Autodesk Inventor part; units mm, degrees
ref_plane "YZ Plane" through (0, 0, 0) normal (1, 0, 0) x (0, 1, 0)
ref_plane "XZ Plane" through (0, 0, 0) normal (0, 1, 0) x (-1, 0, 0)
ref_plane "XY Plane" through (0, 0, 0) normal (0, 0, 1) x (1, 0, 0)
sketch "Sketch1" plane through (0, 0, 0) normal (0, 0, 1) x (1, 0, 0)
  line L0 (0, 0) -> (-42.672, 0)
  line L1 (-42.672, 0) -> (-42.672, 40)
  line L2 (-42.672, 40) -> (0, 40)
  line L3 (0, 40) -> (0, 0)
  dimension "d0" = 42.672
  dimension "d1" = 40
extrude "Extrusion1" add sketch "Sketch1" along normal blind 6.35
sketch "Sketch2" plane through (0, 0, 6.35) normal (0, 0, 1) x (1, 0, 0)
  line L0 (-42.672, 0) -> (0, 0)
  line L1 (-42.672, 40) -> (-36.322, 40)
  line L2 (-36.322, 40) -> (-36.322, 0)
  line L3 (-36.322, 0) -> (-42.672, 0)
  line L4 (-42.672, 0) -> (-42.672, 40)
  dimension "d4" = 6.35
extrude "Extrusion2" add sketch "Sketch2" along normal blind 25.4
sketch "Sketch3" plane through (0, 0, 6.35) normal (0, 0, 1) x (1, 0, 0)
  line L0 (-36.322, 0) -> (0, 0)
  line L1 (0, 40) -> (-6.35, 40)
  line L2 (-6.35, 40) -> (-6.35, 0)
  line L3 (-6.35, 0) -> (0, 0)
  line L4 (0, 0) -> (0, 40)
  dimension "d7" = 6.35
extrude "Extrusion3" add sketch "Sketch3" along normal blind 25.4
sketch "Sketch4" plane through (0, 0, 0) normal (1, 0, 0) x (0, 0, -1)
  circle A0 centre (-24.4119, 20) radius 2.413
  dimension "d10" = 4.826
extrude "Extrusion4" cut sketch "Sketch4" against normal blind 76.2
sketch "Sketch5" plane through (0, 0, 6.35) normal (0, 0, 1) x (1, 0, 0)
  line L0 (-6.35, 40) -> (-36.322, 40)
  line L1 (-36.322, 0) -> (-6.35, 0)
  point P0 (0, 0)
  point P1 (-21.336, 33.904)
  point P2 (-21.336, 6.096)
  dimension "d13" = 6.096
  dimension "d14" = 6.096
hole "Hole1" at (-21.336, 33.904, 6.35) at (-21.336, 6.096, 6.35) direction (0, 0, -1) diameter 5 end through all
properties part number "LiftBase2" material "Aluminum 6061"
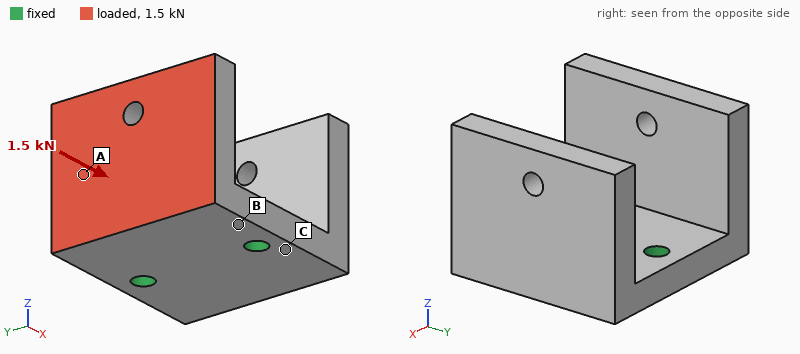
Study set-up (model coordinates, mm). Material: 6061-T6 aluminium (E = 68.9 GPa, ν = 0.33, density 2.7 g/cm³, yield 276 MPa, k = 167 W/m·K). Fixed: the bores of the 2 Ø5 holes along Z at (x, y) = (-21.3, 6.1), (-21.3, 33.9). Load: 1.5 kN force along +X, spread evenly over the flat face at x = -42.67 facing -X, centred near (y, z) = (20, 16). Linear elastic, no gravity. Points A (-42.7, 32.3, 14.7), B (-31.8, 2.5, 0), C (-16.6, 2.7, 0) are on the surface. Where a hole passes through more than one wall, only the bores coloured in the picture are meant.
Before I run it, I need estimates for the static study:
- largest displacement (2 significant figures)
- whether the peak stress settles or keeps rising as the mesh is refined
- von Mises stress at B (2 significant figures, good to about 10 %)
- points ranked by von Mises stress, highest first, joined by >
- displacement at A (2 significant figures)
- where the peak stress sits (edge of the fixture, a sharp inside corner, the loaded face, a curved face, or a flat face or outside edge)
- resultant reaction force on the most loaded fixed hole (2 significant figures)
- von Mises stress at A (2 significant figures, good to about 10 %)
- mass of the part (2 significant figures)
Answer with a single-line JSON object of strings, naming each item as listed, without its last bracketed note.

{"largest displacement": "0.22 mm", "whether the peak stress settles or keeps rising as the mesh is refined": "keeps rising", "von Mises stress at B": "68 MPa", "points ranked by von Mises stress, highest first, joined by >": "B > A > C", "displacement at A": "0.11 mm", "where the peak stress sits": "edge of the fixture", "resultant reaction force on the most loaded fixed hole": "760 N", "von Mises stress at A": "24 MPa", "mass of the part": "63 g"}
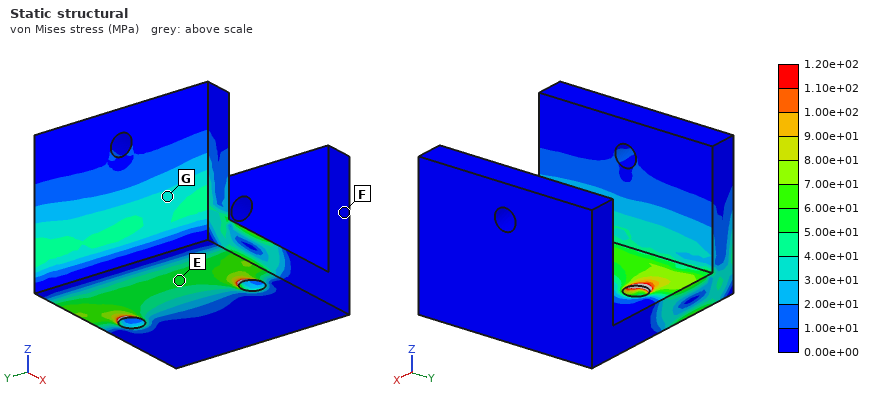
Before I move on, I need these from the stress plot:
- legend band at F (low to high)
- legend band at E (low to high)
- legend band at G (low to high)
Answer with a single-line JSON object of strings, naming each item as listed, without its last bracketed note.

{"legend band at F": "0.00e+00 to 1.00e+01 MPa", "legend band at E": "5.00e+01 to 6.00e+01 MPa", "legend band at G": "3.00e+01 to 4.00e+01 MPa"}
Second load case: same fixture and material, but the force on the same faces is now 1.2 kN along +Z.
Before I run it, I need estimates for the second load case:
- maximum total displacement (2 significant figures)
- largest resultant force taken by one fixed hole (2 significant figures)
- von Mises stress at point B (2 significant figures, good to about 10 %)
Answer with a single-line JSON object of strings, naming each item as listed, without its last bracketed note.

{"maximum total displacement": "0.16 mm", "largest resultant force taken by one fixed hole": "600 N", "von Mises stress at point B": "53 MPa"}
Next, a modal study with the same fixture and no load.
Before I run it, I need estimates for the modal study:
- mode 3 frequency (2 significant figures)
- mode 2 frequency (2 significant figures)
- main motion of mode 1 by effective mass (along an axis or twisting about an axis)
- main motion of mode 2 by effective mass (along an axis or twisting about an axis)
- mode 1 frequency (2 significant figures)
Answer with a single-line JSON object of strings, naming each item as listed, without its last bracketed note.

{"mode 3 frequency": "5800 Hz", "mode 2 frequency": "3300 Hz", "main motion of mode 1 by effective mass": "along X", "main motion of mode 2 by effective mass": "along Z", "mode 1 frequency": "3000 Hz"}
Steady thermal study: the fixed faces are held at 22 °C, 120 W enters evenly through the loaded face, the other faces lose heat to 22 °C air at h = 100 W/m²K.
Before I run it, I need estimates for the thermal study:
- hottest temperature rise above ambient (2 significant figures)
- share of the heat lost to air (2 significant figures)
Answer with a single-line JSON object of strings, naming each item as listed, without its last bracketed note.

{"hottest temperature rise above ambient": "74 K", "share of the heat lost to air": "14 %"}
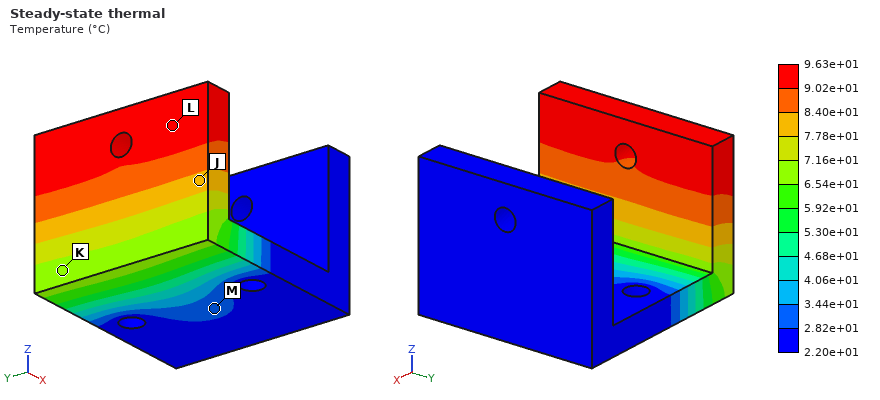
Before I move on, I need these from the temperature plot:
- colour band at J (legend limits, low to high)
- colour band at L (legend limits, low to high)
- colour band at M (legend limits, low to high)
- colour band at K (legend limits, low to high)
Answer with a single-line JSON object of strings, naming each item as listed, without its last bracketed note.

{"colour band at J": "7.78e+01 to 8.40e+01 °C", "colour band at L": "9.02e+01 to 9.63e+01 °C", "colour band at M": "2.82e+01 to 3.44e+01 °C", "colour band at K": "6.54e+01 to 7.16e+01 °C"}
